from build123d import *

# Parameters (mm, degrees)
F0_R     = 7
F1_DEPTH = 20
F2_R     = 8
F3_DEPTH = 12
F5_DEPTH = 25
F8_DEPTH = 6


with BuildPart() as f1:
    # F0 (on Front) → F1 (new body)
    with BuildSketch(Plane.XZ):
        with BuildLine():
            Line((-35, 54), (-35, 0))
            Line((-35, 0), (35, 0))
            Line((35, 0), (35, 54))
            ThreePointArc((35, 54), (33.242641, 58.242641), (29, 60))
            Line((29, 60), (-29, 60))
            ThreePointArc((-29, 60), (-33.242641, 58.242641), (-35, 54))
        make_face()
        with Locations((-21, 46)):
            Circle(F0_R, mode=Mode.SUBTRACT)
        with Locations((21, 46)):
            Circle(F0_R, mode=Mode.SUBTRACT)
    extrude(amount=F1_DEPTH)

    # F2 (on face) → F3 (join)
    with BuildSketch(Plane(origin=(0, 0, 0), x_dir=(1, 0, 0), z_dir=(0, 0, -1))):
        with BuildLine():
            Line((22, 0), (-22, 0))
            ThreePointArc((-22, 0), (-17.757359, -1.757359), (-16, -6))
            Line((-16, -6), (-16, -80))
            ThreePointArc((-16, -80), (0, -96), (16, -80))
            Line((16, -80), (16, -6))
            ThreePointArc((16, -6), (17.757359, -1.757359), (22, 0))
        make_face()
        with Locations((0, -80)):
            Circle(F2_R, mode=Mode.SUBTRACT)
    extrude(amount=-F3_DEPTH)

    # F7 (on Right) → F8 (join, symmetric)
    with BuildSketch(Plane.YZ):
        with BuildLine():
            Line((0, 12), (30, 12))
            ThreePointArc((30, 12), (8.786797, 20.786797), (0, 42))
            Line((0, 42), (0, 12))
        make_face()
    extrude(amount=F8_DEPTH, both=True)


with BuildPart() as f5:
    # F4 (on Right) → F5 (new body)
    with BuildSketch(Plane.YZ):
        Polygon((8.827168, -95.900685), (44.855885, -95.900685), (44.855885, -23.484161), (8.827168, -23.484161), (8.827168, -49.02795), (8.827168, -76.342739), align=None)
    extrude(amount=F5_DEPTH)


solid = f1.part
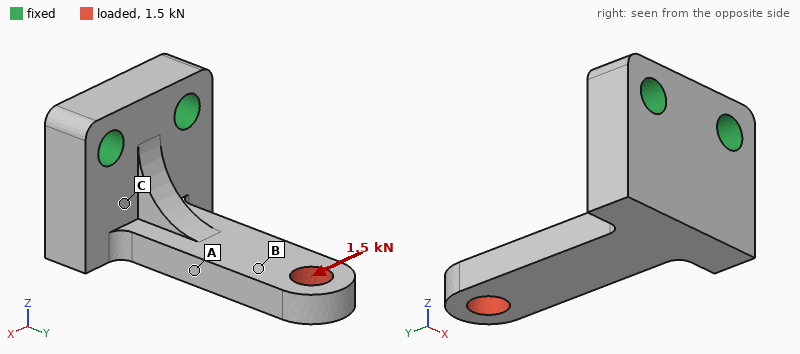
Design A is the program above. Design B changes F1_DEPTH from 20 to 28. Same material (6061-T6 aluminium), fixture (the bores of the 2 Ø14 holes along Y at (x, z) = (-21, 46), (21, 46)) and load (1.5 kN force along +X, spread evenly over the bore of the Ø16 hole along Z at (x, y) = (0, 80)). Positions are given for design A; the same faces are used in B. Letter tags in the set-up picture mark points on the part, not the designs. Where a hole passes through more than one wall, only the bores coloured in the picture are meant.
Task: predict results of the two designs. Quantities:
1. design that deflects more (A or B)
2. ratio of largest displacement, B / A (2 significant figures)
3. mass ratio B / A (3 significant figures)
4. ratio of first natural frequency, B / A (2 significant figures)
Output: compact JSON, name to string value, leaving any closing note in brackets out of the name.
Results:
{"design that deflects more": "A", "ratio of largest displacement, B / A": "0.86", "mass ratio B / A": "1.27", "ratio of first natural frequency, B / A": "1.1"}
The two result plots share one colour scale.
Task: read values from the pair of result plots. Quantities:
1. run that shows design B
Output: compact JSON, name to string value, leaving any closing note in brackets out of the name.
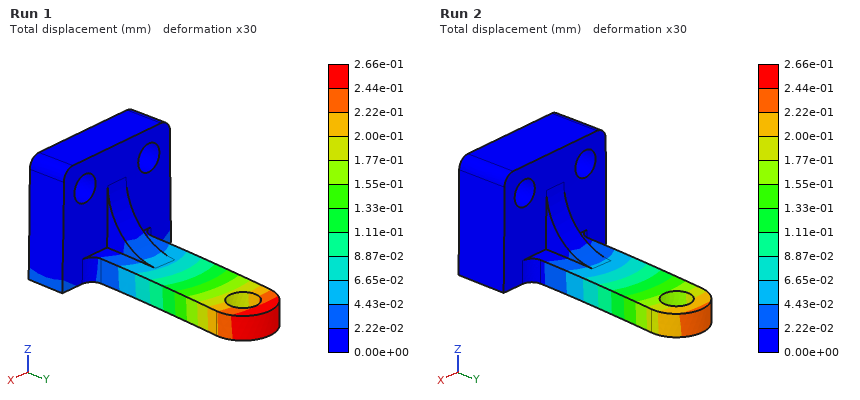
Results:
{"run that shows design B": "Run 2"}
